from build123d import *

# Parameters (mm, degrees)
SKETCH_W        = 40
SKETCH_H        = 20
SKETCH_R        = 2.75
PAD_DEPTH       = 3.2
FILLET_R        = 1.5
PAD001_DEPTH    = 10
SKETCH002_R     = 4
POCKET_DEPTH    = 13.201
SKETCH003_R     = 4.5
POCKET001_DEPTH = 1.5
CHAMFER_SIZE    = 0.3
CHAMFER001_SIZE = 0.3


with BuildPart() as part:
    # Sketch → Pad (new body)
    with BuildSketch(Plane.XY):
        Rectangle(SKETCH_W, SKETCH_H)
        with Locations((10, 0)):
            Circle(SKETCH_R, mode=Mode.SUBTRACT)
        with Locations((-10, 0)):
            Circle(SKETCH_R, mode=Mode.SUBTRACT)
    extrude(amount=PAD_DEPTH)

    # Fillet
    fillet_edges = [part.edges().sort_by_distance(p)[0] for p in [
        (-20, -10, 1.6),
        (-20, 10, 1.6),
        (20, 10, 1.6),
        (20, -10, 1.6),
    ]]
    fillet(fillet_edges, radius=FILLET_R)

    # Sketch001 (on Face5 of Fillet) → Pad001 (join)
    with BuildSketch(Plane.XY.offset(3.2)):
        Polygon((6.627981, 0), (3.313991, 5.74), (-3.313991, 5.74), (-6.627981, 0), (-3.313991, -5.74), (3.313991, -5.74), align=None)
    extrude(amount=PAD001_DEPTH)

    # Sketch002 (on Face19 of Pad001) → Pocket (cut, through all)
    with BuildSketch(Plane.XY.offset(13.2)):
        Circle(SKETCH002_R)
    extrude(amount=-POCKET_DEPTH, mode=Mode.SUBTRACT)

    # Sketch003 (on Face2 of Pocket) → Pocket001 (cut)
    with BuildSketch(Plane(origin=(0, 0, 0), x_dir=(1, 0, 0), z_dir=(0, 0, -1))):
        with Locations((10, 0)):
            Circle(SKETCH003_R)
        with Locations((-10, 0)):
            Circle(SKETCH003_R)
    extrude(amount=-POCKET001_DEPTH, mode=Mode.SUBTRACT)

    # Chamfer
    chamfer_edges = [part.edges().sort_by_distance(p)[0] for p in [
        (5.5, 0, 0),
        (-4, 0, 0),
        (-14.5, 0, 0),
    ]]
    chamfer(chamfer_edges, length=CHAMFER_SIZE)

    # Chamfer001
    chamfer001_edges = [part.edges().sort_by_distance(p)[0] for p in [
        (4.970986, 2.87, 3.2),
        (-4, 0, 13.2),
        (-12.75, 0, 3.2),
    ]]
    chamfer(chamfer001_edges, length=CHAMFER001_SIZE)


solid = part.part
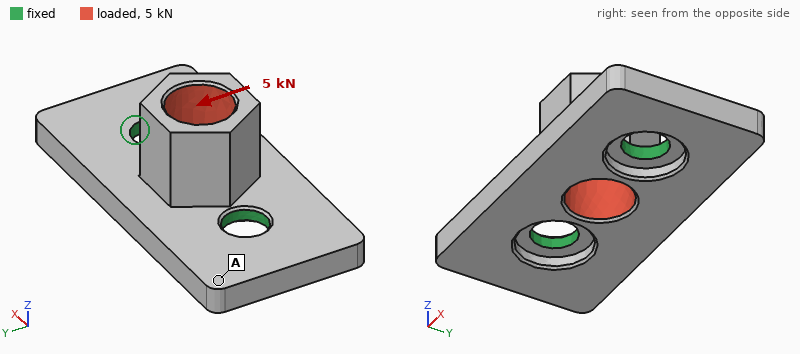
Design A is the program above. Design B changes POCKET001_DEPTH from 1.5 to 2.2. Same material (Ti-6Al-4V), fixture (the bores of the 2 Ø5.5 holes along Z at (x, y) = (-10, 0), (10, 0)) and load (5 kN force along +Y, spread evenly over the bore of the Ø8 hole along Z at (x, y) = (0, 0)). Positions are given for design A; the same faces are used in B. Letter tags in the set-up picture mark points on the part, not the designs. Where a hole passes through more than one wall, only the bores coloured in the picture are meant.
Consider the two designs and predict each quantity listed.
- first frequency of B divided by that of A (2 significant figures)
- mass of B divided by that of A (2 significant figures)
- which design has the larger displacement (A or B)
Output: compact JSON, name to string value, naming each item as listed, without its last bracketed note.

{"first frequency of B divided by that of A": "0.68", "mass of B divided by that of A": "0.98", "which design has the larger displacement": "B"}
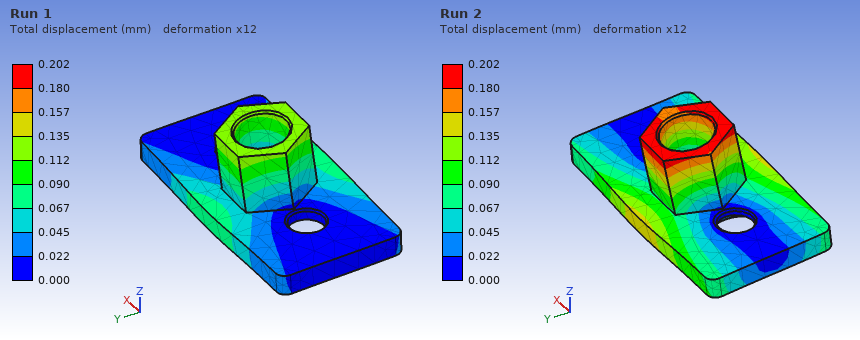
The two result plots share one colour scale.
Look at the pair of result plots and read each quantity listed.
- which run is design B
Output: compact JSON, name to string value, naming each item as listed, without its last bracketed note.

{"which run is design B": "Run 2"}
